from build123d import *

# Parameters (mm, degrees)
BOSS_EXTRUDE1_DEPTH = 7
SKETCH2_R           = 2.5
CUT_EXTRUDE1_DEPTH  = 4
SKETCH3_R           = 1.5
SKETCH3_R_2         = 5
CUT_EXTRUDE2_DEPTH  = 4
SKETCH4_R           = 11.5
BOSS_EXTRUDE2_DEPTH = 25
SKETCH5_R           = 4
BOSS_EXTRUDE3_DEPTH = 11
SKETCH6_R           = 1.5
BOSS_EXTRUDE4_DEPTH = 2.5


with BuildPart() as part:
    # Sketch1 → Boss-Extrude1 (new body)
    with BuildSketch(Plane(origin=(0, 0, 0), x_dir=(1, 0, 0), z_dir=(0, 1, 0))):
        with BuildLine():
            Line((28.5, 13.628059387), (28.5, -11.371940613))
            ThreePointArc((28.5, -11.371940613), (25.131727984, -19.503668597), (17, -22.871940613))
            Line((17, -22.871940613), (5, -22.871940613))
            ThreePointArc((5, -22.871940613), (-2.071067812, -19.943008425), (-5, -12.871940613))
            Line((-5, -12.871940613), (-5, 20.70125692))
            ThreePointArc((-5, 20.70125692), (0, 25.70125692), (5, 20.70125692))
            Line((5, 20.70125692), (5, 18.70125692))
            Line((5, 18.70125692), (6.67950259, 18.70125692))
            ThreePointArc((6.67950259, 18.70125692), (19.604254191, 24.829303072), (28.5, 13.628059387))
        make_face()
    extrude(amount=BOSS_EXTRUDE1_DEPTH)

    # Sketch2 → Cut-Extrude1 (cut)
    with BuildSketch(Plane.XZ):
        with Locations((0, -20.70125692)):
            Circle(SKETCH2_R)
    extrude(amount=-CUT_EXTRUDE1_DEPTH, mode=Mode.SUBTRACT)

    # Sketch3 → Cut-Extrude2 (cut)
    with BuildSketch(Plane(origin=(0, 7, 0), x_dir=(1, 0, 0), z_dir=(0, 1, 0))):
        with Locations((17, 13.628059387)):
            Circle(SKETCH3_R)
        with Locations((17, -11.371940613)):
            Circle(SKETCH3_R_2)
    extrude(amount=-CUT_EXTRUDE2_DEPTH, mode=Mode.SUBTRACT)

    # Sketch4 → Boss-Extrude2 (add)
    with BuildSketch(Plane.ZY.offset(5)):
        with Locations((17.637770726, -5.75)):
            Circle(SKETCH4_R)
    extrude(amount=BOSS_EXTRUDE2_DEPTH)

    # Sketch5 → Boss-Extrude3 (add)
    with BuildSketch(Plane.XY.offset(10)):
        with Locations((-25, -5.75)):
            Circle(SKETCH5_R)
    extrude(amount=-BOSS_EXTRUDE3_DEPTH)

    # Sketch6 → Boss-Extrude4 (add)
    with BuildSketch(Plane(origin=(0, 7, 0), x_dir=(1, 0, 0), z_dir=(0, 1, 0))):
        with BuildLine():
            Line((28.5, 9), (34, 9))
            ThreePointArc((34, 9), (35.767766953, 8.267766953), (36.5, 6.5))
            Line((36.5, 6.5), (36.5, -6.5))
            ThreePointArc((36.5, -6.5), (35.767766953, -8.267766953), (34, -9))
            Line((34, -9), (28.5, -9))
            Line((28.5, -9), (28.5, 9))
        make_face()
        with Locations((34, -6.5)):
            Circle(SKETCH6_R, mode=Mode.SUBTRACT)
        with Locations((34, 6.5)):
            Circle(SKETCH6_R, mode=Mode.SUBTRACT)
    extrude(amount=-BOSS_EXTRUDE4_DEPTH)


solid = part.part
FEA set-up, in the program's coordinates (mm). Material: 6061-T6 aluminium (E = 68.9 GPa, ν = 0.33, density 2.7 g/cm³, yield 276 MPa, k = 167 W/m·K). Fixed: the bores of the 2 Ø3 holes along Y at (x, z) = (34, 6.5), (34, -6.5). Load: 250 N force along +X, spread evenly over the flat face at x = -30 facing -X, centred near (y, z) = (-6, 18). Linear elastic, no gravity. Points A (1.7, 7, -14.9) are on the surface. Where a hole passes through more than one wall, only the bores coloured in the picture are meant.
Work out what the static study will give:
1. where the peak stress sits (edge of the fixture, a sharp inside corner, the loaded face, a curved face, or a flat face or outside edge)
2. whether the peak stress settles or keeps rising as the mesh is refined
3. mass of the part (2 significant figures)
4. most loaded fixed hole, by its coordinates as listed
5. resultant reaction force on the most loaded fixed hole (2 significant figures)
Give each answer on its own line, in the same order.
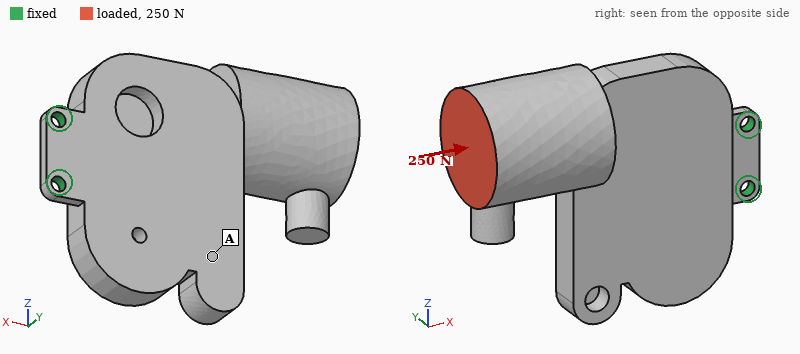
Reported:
edge of the fixture
keeps rising
57 g
(34, 6.5)
450 N
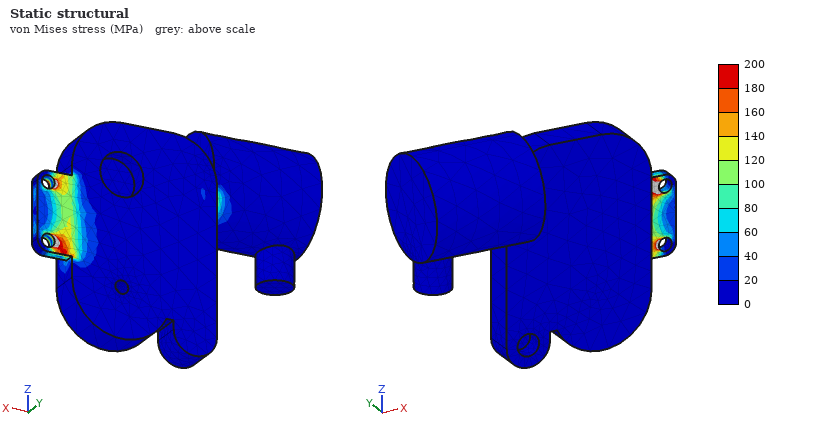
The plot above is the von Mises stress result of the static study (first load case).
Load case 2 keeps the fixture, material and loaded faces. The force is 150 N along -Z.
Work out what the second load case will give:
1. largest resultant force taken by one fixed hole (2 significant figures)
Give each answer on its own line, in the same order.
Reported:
710 N
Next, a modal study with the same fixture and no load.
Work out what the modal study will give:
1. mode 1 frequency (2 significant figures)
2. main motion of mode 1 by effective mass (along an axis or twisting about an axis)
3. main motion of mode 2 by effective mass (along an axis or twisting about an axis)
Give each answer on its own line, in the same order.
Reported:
270 Hz
along Y
along Z
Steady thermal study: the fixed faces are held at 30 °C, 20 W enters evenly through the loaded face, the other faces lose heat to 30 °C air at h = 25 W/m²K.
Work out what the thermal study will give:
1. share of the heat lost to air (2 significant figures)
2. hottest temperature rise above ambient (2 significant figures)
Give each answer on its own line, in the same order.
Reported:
27 %
59 K
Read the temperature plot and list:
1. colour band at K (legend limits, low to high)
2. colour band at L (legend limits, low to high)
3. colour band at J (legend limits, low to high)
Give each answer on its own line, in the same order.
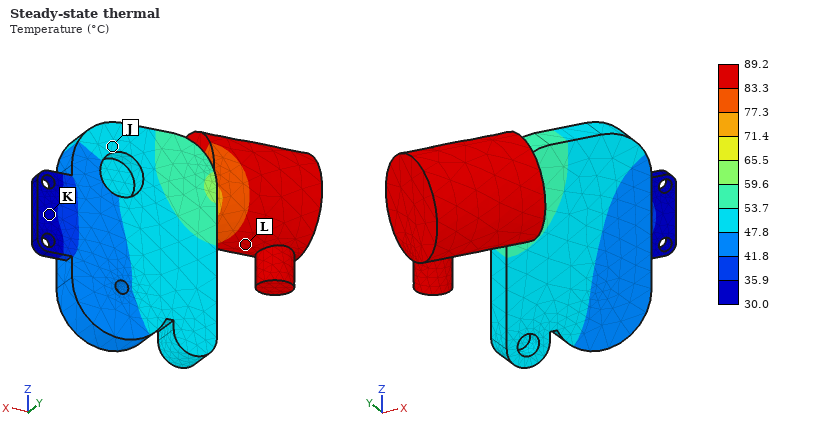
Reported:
30.0 to 35.9 °C
83.3 to 89.2 °C
47.8 to 53.7 °C
